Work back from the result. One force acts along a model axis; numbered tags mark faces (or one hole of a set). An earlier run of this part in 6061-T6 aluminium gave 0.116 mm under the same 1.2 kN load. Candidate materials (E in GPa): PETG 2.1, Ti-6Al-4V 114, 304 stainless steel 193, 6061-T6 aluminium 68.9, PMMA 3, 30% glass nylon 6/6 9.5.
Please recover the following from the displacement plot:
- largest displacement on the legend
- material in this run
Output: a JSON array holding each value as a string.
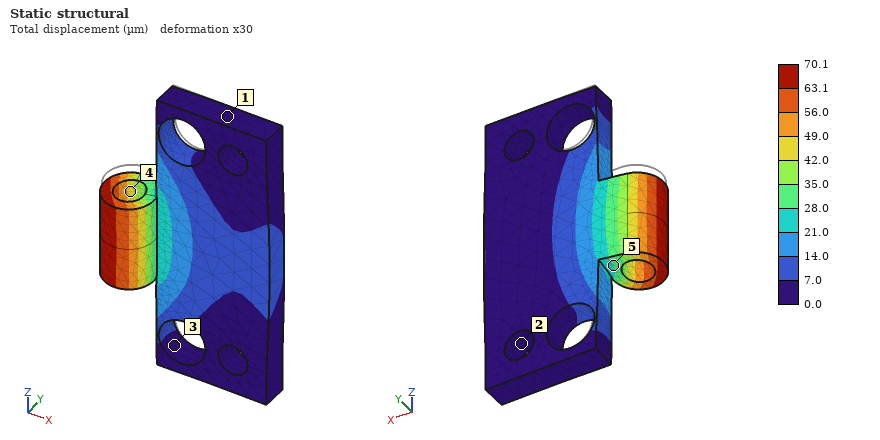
["70.1 µm", "Ti-6Al-4V"]
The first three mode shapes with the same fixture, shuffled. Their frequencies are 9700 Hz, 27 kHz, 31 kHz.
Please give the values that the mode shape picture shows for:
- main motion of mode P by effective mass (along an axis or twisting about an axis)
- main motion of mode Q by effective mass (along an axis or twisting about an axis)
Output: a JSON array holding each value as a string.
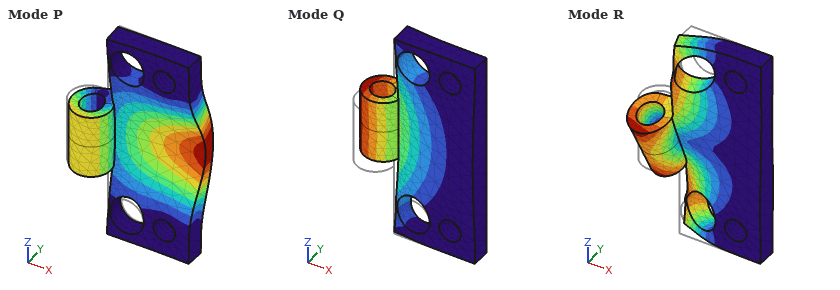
["along Y", "along Y"]
